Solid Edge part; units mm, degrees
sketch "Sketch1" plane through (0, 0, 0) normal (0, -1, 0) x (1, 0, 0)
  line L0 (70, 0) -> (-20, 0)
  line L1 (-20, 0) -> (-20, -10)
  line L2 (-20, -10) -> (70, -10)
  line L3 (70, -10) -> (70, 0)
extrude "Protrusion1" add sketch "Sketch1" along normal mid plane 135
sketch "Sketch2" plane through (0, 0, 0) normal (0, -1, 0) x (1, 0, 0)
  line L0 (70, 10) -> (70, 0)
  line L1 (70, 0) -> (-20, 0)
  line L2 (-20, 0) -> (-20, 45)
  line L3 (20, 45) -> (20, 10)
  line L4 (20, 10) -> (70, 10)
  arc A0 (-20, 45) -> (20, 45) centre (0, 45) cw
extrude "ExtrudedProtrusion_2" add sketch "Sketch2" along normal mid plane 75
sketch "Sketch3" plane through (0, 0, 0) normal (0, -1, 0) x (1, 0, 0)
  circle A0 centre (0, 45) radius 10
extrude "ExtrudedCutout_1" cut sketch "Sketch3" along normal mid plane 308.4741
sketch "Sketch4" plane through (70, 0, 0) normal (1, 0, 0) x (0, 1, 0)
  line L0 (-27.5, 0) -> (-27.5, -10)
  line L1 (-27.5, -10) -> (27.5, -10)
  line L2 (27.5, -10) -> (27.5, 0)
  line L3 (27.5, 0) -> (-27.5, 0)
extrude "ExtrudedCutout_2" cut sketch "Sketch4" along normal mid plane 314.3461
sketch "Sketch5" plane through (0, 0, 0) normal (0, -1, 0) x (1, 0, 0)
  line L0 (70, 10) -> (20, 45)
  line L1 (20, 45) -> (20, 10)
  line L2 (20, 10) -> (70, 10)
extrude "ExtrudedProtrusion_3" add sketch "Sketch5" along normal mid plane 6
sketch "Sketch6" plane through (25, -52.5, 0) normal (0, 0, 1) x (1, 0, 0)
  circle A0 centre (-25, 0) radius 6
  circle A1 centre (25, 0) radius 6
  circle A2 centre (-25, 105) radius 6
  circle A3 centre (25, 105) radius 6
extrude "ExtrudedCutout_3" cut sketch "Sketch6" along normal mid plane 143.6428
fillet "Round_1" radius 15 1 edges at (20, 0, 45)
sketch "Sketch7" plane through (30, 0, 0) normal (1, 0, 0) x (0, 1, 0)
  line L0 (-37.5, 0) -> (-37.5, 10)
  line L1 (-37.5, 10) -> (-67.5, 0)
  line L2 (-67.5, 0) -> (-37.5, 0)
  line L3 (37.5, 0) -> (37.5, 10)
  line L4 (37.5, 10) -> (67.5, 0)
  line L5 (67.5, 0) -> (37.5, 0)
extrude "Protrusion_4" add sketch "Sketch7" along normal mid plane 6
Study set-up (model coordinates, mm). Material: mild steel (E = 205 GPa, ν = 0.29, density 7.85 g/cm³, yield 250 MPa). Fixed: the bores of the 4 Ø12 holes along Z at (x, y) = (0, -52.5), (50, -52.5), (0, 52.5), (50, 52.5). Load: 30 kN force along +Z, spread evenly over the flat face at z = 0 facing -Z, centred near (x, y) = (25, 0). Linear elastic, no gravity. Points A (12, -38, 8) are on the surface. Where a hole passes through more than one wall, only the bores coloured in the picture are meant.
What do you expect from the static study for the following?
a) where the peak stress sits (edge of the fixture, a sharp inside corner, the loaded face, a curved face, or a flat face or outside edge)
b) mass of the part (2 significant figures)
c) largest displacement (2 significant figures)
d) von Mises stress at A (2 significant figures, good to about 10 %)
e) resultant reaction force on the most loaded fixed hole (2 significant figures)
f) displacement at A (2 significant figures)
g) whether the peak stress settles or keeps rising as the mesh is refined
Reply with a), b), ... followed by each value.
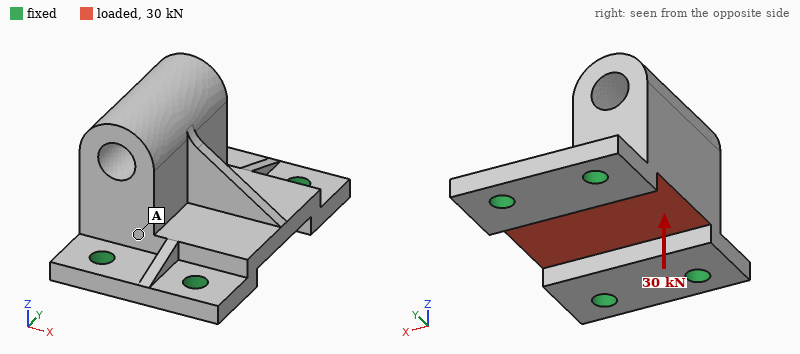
a) edge of the fixture
b) 2.1 kg
c) 40 µm
d) 33 MPa
e) 12 kN
f) 14 µm
g) keeps rising
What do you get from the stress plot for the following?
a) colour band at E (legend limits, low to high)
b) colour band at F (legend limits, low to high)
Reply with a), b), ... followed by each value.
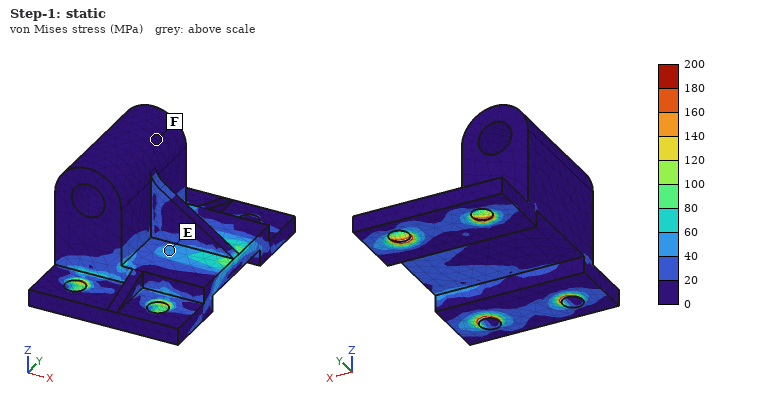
a) 40 to 60 MPa
b) 0 to 20 MPa
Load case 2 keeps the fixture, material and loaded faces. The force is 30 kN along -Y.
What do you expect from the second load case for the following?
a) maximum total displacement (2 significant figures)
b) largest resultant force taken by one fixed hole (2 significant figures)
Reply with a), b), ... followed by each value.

a) 11 µm
b) 7.8 kN
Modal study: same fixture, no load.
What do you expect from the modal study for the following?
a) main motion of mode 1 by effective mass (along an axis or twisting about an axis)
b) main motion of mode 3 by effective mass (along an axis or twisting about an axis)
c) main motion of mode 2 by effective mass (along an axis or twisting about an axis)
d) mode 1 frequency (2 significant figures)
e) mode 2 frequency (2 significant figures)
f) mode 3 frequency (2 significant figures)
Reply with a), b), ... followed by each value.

a) along X
b) along Z
c) along Y
d) 2900 Hz
e) 5000 Hz
f) 5200 Hz
